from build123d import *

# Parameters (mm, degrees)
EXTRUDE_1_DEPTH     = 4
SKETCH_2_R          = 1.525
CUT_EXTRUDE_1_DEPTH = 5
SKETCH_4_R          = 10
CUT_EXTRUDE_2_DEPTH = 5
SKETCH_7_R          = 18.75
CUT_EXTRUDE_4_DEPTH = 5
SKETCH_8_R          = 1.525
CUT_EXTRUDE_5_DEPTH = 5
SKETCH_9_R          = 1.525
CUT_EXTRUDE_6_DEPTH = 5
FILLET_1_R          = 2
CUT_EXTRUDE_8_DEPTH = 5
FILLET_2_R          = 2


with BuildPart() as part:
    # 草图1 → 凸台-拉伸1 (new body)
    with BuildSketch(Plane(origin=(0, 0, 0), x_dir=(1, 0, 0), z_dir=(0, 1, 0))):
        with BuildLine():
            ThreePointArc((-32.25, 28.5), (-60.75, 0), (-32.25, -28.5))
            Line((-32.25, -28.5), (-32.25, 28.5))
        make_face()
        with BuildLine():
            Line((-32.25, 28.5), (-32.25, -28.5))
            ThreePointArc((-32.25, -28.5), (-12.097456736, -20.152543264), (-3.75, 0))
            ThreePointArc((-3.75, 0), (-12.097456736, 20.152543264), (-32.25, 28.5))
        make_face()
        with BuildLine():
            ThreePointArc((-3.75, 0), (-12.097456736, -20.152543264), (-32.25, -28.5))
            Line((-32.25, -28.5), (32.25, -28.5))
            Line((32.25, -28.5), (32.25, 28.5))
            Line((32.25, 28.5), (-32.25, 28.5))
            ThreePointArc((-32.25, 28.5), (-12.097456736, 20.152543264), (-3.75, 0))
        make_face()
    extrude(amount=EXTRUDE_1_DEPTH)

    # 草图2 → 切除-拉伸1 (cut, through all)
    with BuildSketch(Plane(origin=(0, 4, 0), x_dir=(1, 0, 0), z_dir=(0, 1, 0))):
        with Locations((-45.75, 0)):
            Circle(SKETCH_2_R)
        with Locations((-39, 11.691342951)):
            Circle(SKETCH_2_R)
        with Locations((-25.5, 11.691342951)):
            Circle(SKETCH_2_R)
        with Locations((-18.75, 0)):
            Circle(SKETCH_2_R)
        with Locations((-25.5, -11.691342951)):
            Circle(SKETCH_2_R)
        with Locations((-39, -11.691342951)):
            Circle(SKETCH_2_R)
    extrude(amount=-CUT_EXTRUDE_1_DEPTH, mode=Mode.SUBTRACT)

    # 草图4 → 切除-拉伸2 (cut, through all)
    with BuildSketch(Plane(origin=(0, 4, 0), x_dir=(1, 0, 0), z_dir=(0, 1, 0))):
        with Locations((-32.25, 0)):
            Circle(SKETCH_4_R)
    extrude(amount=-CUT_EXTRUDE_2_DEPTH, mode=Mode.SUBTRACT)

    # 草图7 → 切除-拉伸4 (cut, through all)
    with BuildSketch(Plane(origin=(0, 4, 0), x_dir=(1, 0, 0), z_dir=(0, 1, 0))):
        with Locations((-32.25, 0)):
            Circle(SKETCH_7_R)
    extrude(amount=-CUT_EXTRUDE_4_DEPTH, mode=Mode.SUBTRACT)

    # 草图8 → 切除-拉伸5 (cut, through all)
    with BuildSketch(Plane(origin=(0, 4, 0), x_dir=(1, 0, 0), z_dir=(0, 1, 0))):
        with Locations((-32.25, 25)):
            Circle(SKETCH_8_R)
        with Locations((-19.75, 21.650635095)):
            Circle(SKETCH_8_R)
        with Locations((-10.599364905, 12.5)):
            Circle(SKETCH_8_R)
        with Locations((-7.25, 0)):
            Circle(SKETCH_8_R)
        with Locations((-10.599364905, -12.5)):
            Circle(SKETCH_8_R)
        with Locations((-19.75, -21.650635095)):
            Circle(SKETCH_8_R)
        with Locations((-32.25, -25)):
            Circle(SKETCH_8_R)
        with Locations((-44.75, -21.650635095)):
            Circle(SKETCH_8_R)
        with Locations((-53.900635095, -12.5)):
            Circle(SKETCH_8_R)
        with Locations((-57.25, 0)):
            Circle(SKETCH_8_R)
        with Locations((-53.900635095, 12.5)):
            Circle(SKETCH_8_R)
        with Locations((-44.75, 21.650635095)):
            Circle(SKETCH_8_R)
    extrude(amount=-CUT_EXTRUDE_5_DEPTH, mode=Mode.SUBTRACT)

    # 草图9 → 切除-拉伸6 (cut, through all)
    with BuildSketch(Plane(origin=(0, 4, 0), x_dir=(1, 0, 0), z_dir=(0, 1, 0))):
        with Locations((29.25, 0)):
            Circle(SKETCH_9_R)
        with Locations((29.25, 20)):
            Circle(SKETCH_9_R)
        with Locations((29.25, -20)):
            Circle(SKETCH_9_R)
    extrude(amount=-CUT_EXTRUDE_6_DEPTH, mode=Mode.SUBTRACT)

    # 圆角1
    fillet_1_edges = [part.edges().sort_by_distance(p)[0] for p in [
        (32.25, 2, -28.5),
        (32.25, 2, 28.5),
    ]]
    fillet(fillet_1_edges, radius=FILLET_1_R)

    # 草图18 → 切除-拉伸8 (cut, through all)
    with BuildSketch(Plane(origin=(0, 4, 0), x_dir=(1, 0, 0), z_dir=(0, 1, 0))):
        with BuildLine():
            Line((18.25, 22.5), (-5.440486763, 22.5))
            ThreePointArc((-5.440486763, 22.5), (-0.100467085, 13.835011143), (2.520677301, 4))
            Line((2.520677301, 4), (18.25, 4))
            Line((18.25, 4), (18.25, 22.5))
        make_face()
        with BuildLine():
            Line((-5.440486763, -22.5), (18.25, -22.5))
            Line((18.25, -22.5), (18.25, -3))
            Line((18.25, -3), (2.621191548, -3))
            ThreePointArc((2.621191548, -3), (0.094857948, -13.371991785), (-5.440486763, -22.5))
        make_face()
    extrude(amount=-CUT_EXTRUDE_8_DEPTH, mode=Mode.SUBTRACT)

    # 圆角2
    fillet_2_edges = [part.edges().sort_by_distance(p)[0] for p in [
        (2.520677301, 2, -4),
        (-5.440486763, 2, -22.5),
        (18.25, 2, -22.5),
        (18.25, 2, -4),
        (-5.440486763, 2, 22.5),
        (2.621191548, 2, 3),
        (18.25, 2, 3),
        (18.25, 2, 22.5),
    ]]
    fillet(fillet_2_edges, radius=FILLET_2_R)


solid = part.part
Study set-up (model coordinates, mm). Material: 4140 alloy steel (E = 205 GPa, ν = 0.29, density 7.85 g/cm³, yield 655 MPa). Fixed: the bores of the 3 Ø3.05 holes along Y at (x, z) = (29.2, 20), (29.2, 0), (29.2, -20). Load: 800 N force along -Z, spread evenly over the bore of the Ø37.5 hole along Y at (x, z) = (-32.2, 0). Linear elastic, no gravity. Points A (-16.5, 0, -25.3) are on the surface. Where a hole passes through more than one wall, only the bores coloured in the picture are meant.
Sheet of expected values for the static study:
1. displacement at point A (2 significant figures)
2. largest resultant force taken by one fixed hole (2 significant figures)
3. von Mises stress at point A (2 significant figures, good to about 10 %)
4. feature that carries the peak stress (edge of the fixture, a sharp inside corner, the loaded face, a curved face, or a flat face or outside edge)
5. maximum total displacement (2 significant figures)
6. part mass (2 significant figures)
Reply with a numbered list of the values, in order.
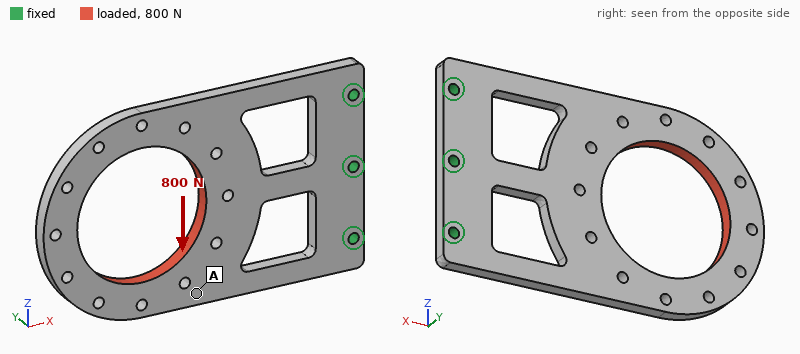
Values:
1. 29 µm
2. 1.2 kN
3. 17 MPa
4. a curved face
5. 51 µm
6. 96 g
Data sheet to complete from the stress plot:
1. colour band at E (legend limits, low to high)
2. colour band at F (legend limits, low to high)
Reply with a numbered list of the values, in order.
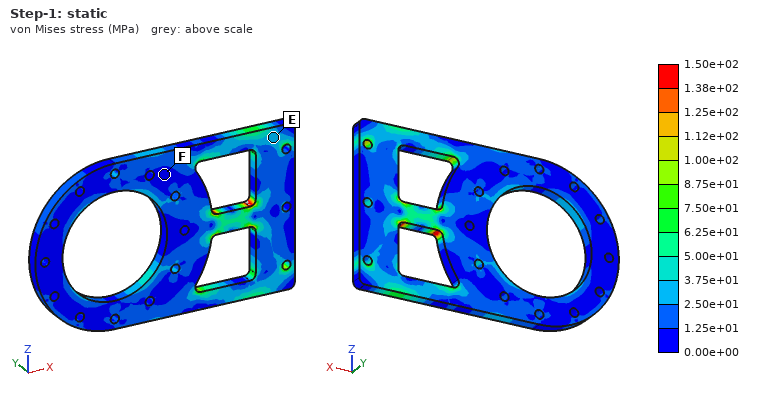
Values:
1. 2.50e+01 to 3.75e+01 MPa
2. 0.00e+00 to 1.25e+01 MPa
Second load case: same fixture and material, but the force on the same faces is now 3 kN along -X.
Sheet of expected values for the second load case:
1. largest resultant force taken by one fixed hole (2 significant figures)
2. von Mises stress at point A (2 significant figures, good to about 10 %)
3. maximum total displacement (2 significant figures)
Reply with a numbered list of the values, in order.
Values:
1. 1.1 kN
2. 30 MPa
3. 20 µm
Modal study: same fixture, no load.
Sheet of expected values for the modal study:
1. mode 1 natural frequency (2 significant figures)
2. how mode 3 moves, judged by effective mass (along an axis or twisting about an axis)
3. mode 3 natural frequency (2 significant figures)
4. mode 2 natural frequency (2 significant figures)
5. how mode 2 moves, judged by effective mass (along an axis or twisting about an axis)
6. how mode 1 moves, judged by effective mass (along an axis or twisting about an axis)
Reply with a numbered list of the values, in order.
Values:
1. 410 Hz
2. along Y
3. 2200 Hz
4. 1300 Hz
5. twisting about X
6. along Y
